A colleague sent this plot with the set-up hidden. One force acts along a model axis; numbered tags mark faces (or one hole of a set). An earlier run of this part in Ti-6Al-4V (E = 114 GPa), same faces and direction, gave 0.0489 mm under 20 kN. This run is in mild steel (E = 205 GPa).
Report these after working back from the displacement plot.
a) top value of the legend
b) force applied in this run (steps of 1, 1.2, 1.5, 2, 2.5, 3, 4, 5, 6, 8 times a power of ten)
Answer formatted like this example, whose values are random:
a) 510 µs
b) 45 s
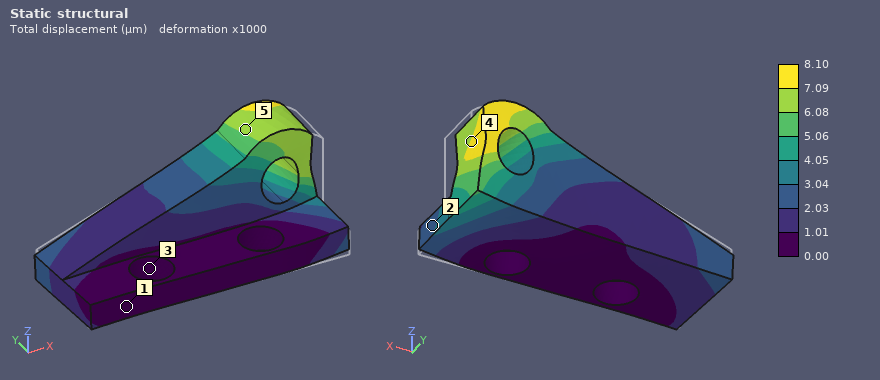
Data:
a) 8.10 µm
b) 6 kN
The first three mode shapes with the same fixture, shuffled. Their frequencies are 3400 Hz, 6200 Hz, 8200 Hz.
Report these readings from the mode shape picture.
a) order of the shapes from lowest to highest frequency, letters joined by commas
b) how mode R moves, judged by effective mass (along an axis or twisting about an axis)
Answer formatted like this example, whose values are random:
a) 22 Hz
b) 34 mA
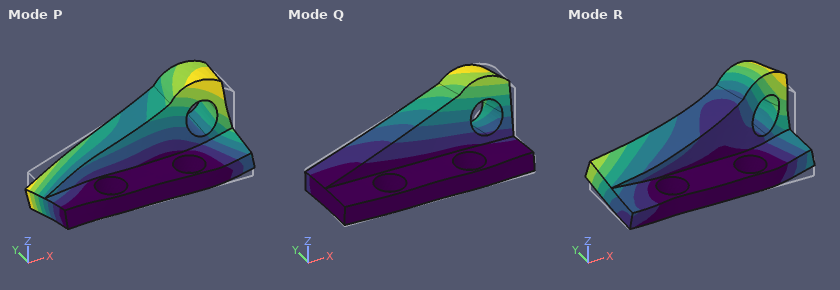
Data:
a) Q, P, R
b) along Z
